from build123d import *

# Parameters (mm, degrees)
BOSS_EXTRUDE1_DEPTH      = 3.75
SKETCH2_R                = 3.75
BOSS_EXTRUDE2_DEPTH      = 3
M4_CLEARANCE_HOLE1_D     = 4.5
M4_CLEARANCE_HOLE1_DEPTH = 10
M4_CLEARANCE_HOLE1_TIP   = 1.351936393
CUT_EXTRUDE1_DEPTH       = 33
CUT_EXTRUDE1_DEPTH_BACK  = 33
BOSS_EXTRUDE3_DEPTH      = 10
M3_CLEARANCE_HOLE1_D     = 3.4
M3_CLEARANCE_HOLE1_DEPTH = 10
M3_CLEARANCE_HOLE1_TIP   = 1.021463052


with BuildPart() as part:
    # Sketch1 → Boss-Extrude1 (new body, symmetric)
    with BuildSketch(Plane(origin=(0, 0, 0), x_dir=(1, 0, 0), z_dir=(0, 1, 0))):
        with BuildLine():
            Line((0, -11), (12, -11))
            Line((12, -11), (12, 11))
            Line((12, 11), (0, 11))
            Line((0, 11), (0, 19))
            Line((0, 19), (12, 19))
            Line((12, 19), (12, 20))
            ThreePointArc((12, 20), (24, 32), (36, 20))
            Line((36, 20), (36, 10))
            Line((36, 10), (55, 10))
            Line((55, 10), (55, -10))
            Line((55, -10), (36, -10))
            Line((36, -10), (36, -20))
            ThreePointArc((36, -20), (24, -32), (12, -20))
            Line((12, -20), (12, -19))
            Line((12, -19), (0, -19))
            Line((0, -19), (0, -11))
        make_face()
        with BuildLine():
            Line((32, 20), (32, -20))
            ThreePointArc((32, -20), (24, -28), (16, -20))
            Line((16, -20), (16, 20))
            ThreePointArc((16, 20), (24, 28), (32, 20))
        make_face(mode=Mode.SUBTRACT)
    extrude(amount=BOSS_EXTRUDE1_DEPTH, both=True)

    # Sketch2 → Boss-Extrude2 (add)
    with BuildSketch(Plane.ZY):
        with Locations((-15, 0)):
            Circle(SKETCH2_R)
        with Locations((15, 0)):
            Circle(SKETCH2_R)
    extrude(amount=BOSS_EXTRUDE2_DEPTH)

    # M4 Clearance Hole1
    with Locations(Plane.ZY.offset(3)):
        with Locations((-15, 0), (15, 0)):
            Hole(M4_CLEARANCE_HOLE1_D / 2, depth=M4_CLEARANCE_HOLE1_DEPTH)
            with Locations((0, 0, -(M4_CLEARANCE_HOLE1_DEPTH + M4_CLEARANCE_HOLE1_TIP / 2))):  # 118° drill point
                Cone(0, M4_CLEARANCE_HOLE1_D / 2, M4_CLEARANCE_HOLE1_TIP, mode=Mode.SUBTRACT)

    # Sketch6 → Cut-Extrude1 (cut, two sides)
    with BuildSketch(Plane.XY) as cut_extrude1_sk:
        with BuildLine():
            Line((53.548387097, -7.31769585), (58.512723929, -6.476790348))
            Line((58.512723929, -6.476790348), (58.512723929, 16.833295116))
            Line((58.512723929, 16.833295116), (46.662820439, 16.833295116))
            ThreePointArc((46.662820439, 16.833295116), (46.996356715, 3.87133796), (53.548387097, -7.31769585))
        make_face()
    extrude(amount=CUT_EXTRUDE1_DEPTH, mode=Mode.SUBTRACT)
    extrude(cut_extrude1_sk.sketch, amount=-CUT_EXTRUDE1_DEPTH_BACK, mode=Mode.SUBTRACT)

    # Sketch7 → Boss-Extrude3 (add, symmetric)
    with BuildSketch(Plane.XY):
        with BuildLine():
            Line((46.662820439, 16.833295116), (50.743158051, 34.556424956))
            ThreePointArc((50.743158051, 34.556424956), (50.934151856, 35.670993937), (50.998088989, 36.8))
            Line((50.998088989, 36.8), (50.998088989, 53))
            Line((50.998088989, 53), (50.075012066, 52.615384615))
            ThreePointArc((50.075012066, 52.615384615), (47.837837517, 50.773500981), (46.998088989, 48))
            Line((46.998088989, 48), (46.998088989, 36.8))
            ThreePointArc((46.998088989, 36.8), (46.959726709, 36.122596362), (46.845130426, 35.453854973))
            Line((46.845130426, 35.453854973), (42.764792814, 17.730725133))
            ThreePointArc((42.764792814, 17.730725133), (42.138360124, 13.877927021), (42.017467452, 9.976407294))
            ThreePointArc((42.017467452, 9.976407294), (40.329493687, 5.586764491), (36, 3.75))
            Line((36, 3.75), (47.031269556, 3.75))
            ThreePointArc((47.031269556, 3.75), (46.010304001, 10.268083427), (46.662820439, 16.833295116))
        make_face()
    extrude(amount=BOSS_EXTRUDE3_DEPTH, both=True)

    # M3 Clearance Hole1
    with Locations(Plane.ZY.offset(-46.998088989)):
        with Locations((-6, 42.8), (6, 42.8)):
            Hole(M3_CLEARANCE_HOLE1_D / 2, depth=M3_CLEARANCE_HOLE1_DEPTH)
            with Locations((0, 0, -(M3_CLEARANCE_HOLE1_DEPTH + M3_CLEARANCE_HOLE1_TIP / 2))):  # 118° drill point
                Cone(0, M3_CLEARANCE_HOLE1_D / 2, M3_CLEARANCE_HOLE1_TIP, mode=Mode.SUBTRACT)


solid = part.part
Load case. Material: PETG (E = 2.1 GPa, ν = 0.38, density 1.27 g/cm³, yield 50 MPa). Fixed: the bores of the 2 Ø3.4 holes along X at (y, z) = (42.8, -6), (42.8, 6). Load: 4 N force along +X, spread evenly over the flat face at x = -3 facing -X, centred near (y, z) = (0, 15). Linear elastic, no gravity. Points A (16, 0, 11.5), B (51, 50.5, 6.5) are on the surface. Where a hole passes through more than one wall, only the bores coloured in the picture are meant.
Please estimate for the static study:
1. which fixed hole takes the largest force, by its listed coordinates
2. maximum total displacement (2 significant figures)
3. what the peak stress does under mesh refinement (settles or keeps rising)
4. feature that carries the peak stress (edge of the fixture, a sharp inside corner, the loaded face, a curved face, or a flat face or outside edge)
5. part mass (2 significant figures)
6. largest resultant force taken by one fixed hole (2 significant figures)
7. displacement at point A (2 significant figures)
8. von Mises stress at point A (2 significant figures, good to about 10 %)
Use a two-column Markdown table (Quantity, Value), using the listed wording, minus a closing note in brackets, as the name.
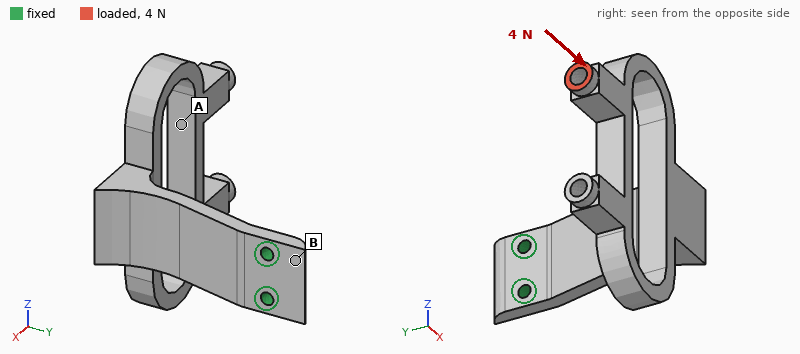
| Quantity | Value |
|---|---|
| which fixed hole takes the largest force, by its listed coordinates | (42.8, 6) |
| maximum total displacement | 1.1 mm |
| what the peak stress does under mesh refinement | keeps rising |
| feature that carries the peak stress | edge of the fixture |
| part mass | 15 g |
| largest resultant force taken by one fixed hole | 6.2 N |
| displacement at point A | 0.79 mm |
| von Mises stress at point A | 0.84 MPa |
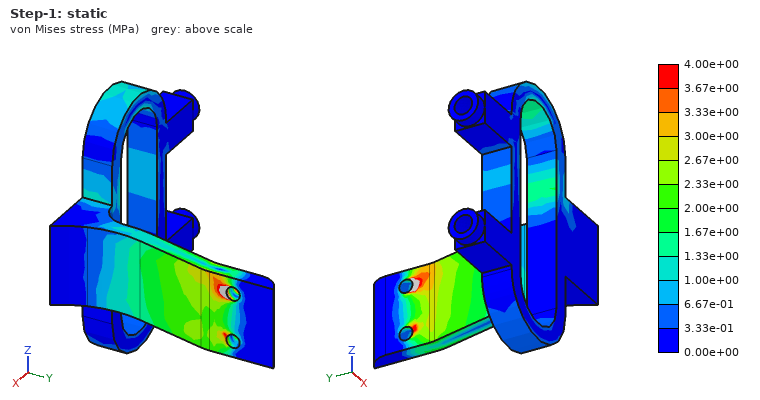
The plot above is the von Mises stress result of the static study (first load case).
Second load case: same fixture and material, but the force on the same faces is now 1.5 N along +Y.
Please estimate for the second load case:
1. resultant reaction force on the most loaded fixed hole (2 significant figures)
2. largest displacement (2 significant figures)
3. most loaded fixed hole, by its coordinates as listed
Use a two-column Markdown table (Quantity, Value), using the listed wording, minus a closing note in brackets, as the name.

| Quantity | Value |
|---|---|
| resultant reaction force on the most loaded fixed hole | 2.5 N |
| largest displacement | 1.0 mm |
| most loaded fixed hole, by its coordinates as listed | (42.8, 6) |
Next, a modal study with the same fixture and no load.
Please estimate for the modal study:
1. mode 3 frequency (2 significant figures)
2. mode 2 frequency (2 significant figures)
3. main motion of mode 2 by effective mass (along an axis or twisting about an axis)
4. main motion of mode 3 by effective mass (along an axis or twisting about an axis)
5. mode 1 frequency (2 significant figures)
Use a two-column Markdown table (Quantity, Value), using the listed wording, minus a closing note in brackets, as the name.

| Quantity | Value |
|---|---|
| mode 3 frequency | 310 Hz |
| mode 2 frequency | 170 Hz |
| main motion of mode 2 by effective mass | along Z |
| main motion of mode 3 by effective mass | along X |
| mode 1 frequency | 110 Hz |
